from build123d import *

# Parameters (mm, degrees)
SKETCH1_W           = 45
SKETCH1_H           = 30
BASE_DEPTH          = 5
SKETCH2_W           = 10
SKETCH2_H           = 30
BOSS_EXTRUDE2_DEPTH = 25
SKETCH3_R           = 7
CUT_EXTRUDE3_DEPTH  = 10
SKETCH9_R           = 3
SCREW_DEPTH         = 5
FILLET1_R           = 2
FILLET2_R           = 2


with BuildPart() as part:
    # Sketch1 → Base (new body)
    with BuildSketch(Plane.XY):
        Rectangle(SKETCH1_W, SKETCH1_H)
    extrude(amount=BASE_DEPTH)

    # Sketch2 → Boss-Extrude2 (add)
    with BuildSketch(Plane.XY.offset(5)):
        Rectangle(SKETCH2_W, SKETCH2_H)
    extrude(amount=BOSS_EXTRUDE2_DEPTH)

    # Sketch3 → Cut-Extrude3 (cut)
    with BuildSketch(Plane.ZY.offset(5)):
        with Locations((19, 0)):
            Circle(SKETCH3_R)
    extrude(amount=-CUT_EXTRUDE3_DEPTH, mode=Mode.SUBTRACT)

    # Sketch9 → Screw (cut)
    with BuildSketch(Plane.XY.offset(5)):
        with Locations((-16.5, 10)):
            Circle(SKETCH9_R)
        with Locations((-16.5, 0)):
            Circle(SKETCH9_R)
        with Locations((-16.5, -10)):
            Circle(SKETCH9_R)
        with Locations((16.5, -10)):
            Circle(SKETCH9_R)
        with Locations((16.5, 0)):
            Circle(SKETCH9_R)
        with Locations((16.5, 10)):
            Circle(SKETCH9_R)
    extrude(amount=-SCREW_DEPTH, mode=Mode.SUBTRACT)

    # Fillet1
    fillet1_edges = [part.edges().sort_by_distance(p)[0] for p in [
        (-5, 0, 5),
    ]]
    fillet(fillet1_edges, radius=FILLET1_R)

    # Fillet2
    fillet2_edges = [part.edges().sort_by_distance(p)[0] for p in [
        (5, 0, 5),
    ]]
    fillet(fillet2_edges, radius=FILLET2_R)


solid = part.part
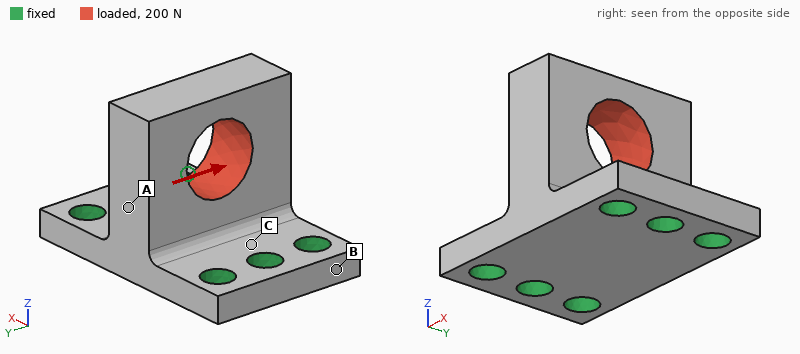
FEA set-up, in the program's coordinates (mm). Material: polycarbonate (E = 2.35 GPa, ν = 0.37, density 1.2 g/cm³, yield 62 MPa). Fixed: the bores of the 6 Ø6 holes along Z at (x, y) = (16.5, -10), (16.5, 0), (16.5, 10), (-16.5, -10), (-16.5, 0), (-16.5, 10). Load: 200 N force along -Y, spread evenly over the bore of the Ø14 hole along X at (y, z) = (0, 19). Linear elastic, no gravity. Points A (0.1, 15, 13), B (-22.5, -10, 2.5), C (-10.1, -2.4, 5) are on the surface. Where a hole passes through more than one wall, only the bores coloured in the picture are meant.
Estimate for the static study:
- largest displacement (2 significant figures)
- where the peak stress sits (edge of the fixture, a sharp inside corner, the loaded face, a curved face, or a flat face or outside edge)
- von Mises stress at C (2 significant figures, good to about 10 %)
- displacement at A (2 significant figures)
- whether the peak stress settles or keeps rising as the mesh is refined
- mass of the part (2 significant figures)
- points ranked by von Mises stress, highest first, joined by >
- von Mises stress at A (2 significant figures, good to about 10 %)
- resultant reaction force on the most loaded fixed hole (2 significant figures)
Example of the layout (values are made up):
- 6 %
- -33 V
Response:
- 0.19 mm
- edge of the fixture
- 3.9 MPa
- 0.098 mm
- keeps rising
- 14 g
- C > A > B
- 2.0 MPa
- 92 N
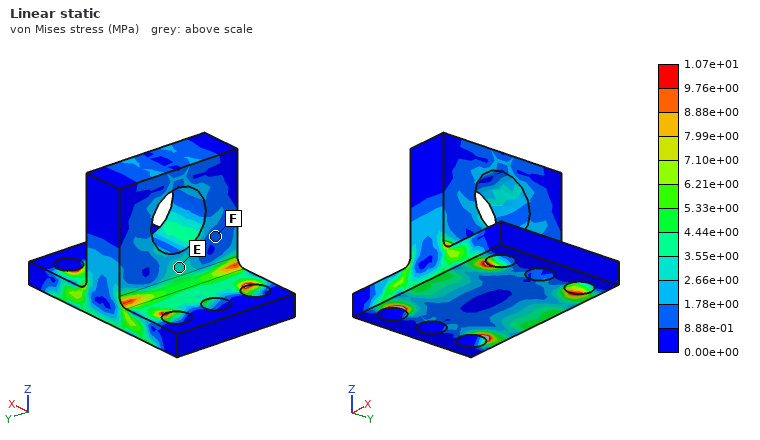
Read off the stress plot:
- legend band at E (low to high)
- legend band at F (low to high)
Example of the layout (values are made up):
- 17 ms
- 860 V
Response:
- 2.66e+00 to 3.55e+00 MPa
- 8.88e-01 to 1.78e+00 MPa
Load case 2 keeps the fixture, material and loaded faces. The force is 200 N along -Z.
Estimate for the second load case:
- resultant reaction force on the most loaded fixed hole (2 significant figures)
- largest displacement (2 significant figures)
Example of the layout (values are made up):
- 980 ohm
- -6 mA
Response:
- 37 N
- 40 µm
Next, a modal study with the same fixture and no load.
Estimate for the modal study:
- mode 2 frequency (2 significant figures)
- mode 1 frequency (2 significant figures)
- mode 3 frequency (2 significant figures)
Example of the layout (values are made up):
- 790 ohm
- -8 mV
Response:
- 2400 Hz
- 2300 Hz
- 4200 Hz
